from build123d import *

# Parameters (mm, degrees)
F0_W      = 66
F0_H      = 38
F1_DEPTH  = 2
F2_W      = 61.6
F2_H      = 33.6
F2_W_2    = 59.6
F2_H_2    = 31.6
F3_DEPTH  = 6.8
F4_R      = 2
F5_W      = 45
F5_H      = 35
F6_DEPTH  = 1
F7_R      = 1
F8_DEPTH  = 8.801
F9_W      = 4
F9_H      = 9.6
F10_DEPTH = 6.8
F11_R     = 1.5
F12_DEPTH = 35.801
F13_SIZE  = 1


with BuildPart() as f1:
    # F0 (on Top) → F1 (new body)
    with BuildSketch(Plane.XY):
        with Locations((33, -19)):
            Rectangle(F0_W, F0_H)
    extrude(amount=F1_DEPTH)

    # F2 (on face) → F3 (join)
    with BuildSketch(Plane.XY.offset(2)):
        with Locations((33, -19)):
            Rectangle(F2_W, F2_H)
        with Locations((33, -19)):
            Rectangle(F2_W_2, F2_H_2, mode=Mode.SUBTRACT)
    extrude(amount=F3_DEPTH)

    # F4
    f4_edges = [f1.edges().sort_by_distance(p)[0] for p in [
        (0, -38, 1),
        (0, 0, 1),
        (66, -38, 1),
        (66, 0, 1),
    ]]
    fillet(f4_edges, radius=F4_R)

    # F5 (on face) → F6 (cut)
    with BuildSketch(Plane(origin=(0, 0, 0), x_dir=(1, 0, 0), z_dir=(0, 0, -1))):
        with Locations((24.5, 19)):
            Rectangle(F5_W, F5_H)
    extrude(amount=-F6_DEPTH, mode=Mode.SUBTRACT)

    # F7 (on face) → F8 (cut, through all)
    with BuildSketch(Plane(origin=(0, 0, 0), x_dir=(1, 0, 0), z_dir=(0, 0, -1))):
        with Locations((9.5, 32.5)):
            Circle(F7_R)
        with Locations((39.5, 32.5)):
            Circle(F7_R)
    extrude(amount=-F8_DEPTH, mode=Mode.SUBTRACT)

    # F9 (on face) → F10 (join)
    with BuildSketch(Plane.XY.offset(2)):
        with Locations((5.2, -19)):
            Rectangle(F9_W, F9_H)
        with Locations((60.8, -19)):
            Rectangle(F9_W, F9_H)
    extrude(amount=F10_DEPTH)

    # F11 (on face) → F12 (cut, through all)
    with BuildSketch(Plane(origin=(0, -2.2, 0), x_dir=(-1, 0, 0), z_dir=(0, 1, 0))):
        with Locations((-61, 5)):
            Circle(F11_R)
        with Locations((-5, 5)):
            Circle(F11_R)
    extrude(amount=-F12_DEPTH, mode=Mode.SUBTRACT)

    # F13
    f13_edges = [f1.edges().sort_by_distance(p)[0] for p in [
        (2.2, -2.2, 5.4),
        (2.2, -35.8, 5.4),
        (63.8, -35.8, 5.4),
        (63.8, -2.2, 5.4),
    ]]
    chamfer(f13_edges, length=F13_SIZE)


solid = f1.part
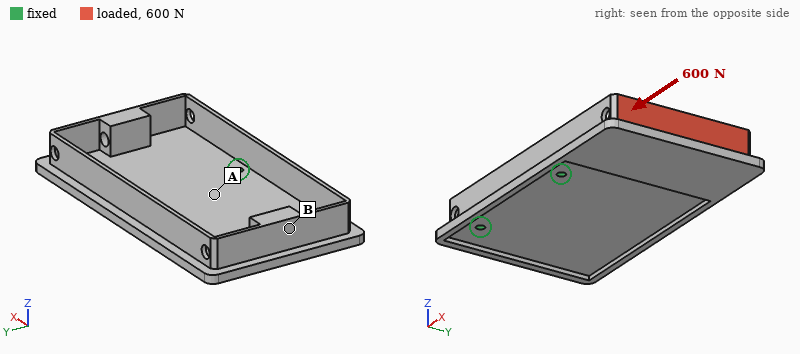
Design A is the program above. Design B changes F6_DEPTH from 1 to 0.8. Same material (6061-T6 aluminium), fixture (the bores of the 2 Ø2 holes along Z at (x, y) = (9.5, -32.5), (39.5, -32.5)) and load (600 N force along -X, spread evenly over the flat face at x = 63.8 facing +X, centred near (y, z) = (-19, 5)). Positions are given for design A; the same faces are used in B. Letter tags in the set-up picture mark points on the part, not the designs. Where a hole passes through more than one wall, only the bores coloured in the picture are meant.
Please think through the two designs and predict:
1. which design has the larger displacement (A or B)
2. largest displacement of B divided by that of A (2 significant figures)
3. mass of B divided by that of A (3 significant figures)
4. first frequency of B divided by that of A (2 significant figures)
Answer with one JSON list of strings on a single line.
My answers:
["A", "0.86", "1.06", "1.2"]
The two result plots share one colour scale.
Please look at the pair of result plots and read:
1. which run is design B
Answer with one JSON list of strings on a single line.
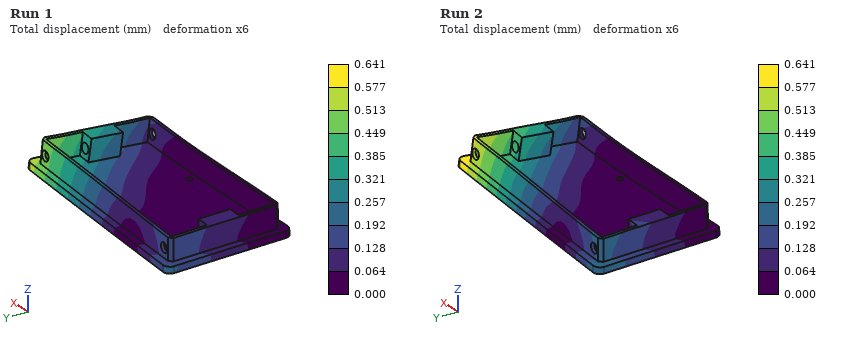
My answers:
["Run 1"]
